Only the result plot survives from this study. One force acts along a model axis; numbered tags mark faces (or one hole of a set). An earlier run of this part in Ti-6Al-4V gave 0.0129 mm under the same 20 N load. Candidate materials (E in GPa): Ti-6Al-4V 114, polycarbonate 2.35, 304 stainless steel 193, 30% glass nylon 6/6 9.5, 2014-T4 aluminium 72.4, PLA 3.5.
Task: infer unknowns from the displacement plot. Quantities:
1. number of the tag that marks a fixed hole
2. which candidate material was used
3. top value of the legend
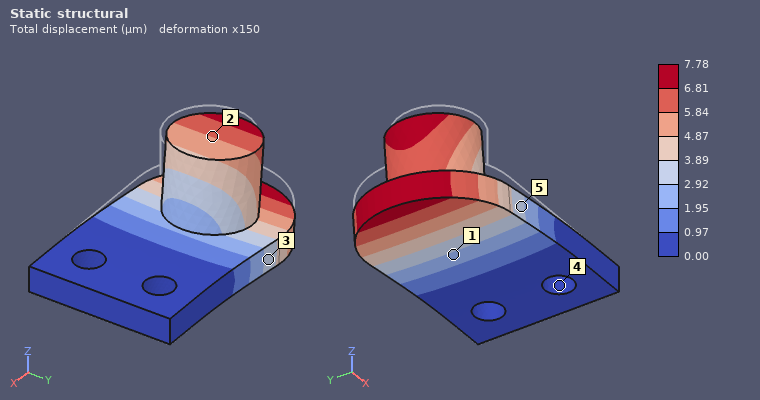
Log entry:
4
304 stainless steel
7.78 µm
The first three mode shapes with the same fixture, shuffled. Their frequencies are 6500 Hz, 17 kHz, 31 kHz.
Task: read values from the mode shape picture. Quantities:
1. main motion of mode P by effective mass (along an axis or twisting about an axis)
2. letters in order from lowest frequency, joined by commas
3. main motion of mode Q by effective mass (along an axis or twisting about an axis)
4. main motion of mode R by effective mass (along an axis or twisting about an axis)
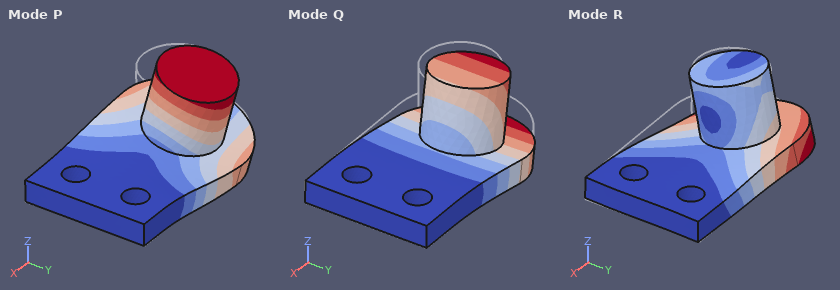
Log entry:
along Y
Q, P, R
along Z
along Y
